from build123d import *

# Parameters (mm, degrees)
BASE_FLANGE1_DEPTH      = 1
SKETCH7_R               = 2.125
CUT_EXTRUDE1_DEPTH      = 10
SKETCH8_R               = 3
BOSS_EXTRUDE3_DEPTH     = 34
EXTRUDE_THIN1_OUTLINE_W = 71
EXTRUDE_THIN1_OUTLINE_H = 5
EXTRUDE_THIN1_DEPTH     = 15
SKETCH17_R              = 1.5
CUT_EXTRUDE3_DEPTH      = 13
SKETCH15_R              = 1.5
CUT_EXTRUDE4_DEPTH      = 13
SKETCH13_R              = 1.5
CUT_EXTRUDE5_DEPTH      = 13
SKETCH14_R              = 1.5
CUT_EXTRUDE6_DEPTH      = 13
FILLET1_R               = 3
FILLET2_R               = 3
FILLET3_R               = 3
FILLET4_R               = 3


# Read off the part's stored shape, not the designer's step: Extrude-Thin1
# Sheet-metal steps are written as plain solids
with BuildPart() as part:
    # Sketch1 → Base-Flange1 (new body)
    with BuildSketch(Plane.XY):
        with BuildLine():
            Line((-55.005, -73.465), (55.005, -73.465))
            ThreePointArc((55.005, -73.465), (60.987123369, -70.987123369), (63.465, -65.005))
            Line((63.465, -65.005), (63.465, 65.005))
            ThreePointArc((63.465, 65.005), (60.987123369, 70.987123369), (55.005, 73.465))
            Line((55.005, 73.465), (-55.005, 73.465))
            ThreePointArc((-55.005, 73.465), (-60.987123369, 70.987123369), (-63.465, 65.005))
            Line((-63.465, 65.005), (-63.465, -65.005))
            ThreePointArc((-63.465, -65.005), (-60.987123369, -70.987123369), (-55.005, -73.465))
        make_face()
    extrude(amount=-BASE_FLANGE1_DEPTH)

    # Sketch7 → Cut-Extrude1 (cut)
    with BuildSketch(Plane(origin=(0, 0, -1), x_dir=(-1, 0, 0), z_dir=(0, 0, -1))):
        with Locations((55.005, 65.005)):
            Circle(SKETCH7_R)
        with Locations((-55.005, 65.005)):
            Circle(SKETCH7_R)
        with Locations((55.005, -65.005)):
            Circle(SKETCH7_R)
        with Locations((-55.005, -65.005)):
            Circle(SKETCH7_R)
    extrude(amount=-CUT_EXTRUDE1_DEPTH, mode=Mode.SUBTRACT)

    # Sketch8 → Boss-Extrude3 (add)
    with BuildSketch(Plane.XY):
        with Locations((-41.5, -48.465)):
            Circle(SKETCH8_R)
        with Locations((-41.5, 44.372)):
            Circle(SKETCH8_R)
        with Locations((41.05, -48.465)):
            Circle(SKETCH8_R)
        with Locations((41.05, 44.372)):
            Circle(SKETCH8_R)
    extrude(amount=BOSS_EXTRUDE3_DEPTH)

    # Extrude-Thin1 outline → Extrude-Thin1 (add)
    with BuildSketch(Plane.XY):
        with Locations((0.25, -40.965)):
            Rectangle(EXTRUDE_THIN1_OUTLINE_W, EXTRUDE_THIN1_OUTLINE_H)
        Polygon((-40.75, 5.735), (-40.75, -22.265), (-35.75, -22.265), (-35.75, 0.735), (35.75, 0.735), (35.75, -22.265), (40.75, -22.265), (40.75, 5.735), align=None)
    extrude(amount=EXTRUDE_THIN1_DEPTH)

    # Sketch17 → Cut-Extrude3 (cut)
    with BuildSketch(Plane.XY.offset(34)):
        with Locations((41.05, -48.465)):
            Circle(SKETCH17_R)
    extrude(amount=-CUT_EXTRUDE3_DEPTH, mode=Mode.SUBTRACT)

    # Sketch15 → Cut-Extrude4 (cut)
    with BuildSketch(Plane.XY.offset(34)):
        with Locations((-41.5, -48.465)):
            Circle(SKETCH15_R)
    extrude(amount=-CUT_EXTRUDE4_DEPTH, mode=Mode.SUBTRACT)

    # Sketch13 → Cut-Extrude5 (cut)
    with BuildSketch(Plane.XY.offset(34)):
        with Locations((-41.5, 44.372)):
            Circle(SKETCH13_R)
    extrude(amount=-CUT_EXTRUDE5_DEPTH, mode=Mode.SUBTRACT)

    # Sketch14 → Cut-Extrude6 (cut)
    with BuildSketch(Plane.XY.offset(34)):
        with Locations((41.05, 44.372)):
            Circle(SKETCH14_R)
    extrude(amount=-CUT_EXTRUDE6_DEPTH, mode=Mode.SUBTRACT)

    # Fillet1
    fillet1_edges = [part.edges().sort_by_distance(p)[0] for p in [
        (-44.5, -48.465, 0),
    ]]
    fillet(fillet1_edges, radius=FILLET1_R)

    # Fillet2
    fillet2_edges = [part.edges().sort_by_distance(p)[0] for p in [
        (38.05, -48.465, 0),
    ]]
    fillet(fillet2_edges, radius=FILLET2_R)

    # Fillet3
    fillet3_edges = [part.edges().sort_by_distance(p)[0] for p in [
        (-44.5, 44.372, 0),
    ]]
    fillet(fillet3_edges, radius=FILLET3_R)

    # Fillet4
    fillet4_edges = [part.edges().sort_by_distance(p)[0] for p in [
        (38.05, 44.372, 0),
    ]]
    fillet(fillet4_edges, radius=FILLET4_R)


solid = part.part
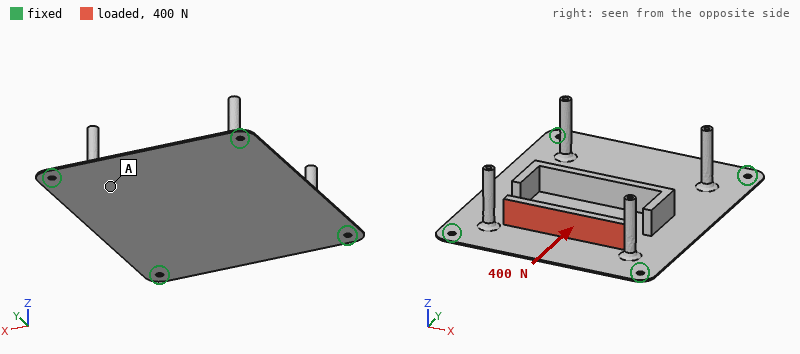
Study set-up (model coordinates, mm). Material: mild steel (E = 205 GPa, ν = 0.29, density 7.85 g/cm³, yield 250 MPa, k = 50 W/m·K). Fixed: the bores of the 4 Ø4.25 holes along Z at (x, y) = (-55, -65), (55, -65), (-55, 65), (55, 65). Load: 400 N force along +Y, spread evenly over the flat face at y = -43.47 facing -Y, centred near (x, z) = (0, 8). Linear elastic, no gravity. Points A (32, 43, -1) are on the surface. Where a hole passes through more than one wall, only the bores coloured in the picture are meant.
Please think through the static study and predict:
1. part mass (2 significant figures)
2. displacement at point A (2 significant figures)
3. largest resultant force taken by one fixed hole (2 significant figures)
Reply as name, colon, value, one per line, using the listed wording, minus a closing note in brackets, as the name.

part mass: 290 g
displacement at point A: 0.14 mm
largest resultant force taken by one fixed hole: 130 N
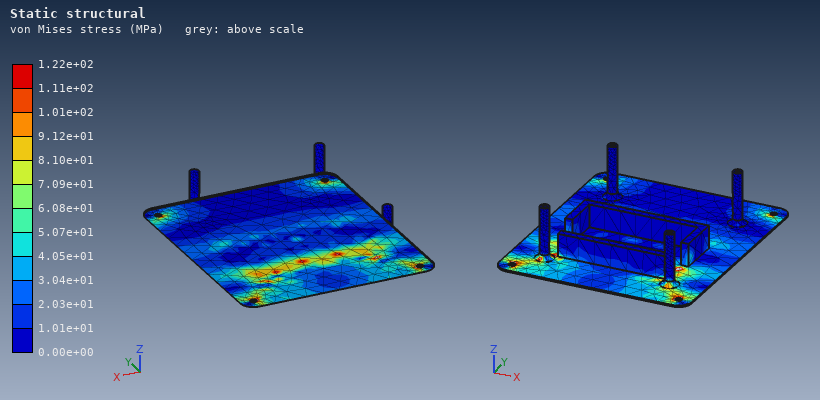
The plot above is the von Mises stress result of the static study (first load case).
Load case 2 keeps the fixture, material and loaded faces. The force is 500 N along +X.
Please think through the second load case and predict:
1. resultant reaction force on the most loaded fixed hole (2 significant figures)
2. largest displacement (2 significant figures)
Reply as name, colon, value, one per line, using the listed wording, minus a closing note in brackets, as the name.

resultant reaction force on the most loaded fixed hole: 210 N
largest displacement: 0.18 mm
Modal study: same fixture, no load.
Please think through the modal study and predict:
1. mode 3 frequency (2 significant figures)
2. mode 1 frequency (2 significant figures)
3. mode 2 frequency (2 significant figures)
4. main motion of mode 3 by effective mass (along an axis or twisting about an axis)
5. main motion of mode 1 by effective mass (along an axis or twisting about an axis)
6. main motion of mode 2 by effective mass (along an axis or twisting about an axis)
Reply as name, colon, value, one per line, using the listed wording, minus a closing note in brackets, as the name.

mode 3 frequency: 420 Hz
mode 1 frequency: 180 Hz
mode 2 frequency: 360 Hz
main motion of mode 3 by effective mass: twisting about X
main motion of mode 1 by effective mass: along Z
main motion of mode 2 by effective mass: twisting about Y
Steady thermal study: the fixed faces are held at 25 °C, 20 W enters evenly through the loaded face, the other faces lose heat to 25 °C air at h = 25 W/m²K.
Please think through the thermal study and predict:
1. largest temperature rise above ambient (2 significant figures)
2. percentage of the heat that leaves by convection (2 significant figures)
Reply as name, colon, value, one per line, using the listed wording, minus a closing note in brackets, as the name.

largest temperature rise above ambient: 63 K
percentage of the heat that leaves by convection: 84 %
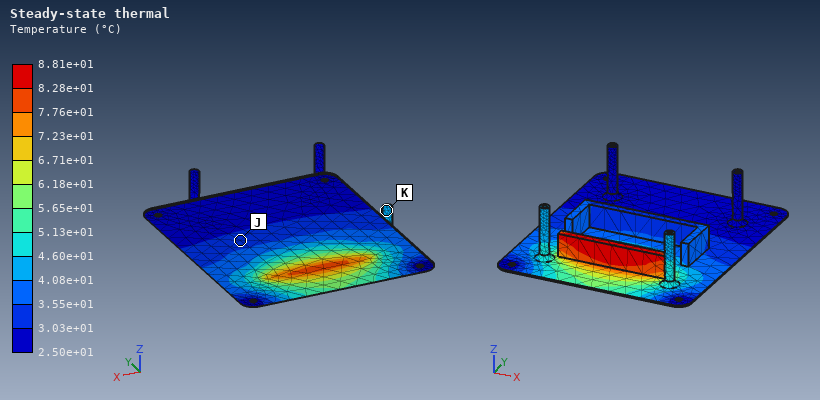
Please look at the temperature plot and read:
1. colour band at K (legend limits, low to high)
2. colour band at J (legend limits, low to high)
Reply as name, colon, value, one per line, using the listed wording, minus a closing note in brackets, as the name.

colour band at K: 4.08e+01 to 4.60e+01 °C
colour band at J: 3.03e+01 to 3.55e+01 °C
